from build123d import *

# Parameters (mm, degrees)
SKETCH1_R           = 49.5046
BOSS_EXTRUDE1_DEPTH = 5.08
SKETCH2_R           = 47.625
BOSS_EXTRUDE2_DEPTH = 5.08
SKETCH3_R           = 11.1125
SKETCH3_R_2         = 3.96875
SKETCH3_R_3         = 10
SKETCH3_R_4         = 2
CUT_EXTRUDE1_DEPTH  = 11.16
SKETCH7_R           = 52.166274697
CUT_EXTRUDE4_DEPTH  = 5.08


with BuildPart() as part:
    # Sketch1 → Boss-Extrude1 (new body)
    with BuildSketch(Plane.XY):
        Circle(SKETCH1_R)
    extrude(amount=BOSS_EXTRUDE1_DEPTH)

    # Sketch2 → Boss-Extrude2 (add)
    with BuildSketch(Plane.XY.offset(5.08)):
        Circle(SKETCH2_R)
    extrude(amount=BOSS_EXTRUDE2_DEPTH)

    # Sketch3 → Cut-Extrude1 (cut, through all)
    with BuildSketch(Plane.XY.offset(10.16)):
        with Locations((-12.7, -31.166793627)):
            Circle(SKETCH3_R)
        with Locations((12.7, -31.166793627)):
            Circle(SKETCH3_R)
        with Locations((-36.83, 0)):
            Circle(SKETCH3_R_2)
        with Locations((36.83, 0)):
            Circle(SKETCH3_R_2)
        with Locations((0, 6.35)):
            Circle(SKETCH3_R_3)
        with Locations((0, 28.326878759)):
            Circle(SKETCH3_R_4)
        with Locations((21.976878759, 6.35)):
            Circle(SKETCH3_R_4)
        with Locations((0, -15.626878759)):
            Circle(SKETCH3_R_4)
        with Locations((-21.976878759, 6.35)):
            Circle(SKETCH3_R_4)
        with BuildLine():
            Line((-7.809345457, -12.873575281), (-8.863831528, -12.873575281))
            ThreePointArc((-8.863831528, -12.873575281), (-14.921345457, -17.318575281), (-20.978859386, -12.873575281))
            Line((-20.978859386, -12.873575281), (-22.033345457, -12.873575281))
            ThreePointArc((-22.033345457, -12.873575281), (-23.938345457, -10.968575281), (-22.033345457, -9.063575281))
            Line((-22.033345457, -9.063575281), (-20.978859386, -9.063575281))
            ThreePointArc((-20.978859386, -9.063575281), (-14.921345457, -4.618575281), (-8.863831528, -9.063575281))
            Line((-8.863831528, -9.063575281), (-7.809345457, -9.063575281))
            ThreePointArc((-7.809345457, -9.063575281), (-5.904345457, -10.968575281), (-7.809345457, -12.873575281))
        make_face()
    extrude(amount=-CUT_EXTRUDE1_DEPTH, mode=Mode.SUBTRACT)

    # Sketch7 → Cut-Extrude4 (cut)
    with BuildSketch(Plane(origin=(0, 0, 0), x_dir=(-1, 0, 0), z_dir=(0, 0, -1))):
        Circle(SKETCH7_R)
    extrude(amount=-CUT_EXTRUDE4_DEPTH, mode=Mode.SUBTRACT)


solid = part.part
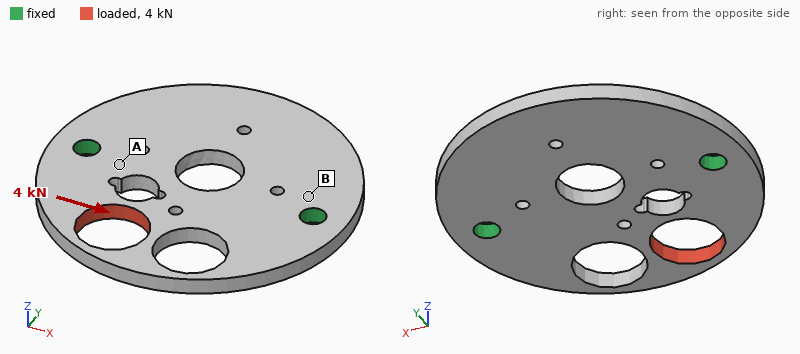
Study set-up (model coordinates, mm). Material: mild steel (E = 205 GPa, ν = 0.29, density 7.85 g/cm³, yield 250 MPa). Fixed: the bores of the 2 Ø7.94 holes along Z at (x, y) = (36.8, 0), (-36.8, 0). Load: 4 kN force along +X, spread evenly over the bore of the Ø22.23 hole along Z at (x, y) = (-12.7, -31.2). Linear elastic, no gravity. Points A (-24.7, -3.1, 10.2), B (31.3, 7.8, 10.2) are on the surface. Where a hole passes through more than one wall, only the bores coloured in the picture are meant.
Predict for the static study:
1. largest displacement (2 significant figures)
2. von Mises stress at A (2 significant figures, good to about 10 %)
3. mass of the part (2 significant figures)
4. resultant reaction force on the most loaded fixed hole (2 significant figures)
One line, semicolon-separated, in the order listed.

26 µm; 26 MPa; 230 g; 2.5 kN
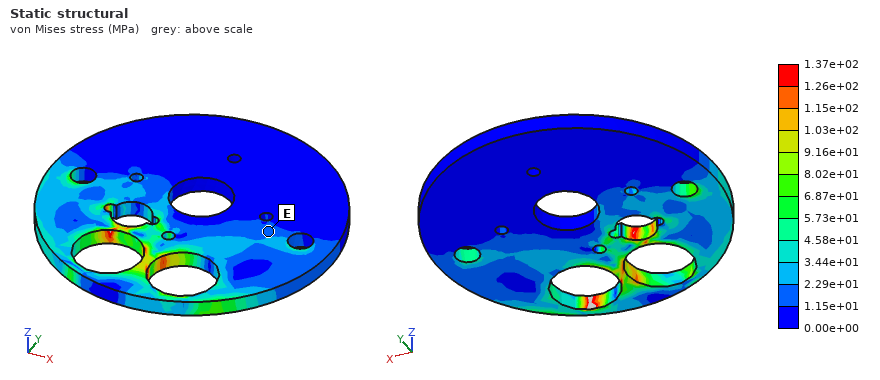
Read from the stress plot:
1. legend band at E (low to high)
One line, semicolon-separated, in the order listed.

1.15e+01 to 2.29e+01 MPa
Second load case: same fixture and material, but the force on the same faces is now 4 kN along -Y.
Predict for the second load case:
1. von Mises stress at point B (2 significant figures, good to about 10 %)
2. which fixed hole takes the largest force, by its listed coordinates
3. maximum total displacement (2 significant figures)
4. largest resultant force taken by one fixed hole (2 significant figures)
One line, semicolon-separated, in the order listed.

11 MPa; (-36.8, 0); 15 µm; 2.8 kN
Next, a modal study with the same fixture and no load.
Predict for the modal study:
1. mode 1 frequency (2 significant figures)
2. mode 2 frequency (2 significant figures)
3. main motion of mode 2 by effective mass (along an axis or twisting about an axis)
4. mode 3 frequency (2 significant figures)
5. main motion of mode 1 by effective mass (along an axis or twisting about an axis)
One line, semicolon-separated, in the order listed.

1900 Hz; 2400 Hz; along Z; 4700 Hz; along Z
